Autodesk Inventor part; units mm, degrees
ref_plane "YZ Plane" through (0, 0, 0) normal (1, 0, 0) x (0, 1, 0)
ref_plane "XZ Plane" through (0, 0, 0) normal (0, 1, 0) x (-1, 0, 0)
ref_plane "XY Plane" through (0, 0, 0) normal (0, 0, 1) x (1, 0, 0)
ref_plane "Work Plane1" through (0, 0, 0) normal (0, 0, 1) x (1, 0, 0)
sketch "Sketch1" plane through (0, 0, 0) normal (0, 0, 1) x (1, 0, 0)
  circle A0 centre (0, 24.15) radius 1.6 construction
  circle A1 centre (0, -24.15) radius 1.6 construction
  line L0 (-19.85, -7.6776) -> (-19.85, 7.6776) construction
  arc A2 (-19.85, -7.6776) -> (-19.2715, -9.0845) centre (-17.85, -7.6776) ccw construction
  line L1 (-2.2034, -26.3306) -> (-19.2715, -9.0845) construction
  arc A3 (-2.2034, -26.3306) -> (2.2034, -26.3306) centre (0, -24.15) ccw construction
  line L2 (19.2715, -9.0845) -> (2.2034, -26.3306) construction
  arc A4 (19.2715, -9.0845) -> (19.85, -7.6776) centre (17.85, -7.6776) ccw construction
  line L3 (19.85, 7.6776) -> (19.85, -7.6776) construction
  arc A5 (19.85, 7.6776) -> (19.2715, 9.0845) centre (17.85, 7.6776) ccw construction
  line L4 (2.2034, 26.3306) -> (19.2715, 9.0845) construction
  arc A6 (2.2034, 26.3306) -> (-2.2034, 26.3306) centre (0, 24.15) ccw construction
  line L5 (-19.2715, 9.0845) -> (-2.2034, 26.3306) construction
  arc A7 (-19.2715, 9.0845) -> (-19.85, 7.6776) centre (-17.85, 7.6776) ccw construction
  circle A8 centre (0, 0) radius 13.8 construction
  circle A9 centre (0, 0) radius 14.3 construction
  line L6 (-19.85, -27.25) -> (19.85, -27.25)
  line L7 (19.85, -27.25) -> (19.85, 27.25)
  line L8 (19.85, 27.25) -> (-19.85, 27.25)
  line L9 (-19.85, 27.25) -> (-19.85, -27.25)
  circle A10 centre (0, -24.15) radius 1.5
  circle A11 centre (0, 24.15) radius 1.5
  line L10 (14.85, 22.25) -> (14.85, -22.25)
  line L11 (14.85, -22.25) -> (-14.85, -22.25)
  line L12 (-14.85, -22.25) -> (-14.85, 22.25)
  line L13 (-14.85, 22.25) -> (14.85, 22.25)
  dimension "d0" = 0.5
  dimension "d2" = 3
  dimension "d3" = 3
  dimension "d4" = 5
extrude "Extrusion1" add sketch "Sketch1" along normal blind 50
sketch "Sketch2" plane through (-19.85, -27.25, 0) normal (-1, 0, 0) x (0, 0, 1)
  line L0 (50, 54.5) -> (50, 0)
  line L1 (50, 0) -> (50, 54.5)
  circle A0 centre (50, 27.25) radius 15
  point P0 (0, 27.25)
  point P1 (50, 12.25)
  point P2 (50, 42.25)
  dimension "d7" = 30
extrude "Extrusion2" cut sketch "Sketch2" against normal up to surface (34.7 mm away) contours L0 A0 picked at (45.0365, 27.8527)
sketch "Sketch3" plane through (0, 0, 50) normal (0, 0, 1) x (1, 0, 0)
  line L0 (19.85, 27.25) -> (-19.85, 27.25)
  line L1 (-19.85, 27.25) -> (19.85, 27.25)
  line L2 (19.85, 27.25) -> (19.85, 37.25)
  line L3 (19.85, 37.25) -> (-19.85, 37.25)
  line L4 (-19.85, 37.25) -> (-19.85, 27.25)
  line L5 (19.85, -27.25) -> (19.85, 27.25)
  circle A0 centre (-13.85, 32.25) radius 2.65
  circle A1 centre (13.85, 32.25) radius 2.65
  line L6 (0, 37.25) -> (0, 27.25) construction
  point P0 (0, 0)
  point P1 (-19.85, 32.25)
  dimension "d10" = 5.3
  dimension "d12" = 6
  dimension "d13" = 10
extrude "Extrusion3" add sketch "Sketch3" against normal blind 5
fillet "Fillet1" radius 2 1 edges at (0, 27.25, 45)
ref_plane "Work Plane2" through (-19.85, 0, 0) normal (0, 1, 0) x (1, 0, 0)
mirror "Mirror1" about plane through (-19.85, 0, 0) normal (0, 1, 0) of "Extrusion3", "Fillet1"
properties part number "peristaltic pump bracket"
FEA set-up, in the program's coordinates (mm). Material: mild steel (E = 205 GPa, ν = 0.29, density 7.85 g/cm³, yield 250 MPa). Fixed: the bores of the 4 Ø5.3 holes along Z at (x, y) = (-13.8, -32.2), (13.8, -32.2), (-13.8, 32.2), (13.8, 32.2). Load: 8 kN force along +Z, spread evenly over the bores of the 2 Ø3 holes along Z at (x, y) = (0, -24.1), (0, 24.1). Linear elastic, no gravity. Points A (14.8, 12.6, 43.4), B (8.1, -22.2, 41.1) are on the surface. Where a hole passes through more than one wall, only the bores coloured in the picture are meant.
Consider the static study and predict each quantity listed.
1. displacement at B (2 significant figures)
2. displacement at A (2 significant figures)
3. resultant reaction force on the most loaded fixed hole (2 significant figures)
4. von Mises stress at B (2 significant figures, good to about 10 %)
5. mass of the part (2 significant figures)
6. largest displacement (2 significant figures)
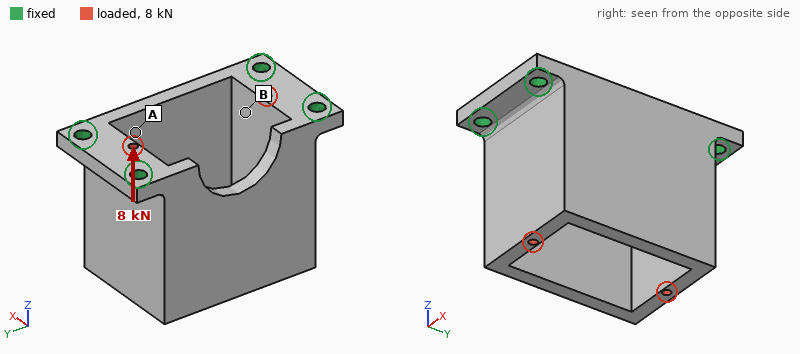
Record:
5.6 µm
5.1 µm
2.1 kN
27 MPa
340 g
7.5 µm
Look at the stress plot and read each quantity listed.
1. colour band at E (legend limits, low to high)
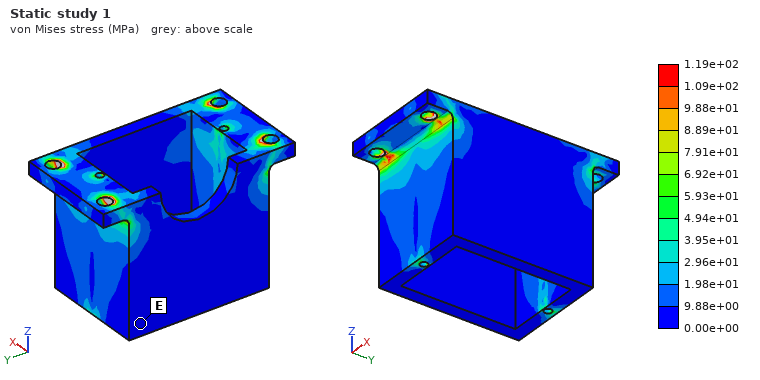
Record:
0.00e+00 to 9.88e+00 MPa
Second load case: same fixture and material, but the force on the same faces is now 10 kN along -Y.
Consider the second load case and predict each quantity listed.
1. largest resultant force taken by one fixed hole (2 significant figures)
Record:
3.2 kN
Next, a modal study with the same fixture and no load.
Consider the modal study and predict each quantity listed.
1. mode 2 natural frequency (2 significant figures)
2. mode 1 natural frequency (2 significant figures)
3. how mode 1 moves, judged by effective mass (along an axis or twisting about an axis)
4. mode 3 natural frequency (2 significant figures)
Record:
6700 Hz
4500 Hz
along X
6900 Hz
